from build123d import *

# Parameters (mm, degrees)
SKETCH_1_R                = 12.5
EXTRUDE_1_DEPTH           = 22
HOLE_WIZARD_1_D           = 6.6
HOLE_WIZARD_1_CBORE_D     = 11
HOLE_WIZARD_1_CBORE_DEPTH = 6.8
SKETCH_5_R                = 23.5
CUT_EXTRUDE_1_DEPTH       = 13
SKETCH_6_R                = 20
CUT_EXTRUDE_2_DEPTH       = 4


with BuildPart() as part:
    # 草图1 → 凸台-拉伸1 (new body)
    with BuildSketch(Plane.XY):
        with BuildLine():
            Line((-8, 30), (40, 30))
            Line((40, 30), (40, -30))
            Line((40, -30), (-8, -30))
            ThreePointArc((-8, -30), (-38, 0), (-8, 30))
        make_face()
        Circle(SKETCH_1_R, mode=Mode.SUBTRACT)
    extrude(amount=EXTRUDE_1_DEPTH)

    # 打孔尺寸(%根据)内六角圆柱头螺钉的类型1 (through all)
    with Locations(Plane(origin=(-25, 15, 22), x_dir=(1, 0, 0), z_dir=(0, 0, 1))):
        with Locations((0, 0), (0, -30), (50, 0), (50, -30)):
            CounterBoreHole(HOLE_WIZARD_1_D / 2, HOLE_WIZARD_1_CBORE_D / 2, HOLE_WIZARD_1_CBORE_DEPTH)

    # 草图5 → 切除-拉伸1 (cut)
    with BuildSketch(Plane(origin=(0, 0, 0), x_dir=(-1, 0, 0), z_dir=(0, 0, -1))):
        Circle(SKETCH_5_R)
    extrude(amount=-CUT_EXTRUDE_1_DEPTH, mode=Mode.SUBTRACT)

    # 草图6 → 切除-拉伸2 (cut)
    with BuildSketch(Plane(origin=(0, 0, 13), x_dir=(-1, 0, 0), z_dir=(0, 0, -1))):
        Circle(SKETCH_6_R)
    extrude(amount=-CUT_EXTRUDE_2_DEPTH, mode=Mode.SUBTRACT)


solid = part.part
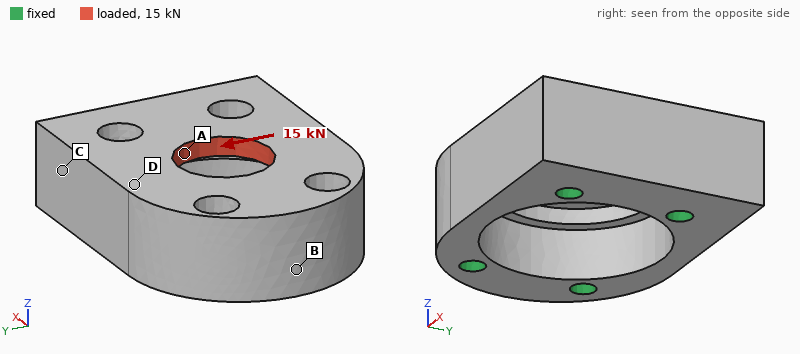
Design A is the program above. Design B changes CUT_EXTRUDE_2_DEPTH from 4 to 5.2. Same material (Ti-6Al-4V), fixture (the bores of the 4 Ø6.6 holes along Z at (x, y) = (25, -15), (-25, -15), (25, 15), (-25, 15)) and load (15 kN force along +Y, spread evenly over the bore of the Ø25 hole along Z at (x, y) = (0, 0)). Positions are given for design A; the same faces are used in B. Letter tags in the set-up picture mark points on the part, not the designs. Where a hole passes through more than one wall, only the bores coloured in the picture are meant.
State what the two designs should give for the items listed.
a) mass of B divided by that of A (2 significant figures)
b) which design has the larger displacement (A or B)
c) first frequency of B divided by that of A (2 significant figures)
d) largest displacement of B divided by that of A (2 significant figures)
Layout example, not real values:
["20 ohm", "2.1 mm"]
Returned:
["0.98", "B", "1.0", "1.2"]
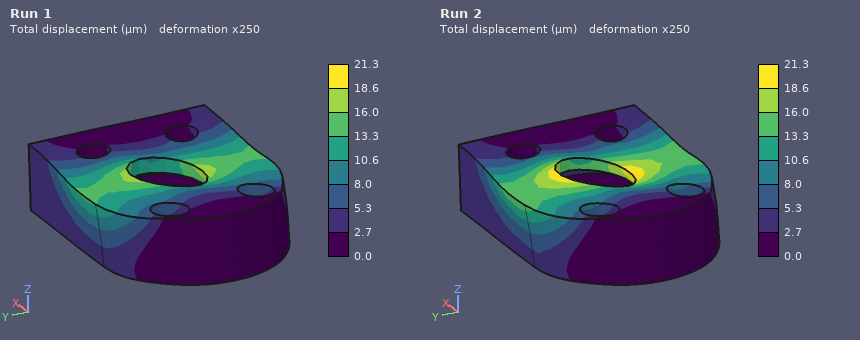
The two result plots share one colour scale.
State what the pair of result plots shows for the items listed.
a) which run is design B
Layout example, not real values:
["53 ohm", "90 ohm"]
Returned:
["Run 2"]
